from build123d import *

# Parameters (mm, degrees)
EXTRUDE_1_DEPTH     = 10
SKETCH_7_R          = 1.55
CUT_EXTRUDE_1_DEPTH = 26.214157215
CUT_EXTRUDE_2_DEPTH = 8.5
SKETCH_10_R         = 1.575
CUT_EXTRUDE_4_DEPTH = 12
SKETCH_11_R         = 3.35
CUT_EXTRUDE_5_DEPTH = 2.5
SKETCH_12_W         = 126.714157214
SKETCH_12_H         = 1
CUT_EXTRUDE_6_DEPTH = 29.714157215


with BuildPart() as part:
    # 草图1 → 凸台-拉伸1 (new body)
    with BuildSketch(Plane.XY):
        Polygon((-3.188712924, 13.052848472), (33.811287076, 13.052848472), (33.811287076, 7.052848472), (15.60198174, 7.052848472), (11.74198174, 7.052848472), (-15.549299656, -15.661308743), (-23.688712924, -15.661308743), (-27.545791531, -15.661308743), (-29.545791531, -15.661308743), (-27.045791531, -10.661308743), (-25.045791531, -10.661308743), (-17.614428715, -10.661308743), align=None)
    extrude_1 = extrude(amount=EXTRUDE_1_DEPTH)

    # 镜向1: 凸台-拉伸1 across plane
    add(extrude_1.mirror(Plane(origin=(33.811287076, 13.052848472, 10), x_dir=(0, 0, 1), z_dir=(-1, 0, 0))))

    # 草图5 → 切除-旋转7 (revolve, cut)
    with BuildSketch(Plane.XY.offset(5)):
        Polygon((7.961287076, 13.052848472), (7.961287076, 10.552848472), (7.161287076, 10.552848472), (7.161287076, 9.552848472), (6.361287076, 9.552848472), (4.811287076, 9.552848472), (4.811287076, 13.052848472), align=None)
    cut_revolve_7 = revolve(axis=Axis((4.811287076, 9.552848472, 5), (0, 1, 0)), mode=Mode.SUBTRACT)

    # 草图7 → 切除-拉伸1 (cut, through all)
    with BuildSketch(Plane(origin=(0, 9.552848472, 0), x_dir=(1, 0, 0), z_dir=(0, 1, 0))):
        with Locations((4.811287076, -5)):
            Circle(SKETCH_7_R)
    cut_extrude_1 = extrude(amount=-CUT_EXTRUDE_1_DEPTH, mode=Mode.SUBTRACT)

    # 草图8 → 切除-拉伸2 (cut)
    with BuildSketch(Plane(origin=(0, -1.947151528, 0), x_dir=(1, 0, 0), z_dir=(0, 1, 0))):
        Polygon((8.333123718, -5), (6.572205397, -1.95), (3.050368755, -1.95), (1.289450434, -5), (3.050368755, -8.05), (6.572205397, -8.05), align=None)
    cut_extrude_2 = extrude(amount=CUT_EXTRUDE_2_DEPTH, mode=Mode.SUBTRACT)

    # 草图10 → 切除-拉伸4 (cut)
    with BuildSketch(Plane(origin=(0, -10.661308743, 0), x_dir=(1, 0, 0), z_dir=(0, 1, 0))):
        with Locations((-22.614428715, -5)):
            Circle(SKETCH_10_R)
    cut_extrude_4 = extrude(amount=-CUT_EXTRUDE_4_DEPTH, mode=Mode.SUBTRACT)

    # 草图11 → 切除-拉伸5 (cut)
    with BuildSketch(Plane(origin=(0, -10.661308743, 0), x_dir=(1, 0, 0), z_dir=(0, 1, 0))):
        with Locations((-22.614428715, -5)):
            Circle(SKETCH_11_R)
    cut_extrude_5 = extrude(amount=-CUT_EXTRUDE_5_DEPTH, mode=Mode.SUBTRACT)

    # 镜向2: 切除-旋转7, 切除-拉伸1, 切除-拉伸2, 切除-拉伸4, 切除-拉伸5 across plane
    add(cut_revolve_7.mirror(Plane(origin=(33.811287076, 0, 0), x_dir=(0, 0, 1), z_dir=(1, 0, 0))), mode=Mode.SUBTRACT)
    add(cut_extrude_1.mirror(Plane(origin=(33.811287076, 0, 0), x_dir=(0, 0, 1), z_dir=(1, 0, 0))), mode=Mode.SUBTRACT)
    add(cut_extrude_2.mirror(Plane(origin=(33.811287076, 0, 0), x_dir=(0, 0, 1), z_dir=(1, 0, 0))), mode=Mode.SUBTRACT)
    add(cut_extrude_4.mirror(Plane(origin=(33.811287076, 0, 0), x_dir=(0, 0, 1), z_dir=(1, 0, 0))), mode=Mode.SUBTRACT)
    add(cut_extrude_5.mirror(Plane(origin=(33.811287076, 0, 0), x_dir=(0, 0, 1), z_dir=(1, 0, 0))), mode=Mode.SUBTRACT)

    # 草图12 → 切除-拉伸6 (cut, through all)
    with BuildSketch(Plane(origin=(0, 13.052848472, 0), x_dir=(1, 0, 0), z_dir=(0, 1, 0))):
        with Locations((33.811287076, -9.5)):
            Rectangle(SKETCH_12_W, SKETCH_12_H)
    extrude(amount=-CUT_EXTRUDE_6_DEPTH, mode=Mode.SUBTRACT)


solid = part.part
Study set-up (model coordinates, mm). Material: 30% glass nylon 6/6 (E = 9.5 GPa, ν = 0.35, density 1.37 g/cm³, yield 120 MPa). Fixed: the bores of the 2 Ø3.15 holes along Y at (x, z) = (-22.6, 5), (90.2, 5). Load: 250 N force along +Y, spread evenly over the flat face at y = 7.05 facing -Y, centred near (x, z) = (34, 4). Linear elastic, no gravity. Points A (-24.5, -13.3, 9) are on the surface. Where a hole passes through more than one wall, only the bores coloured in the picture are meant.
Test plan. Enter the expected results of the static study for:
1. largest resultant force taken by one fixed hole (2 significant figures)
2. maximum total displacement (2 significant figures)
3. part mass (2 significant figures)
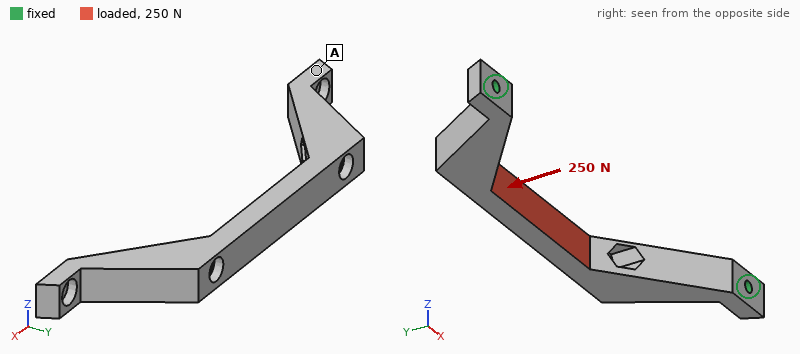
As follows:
230 N
0.17 mm
12 g
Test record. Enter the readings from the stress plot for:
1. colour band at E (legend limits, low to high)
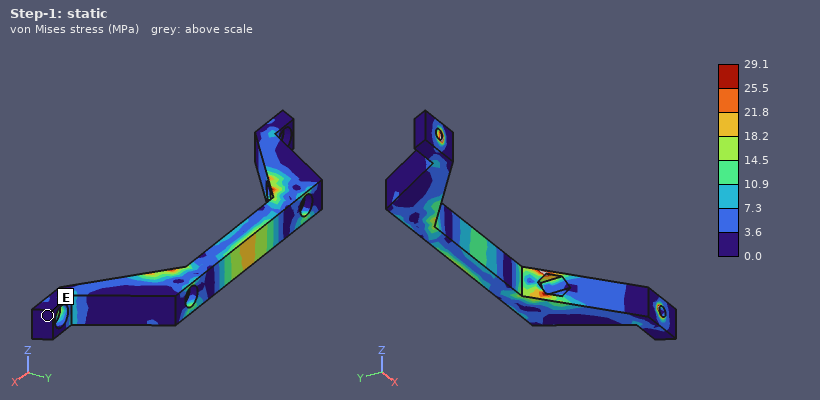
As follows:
0.0 to 3.6 MPa
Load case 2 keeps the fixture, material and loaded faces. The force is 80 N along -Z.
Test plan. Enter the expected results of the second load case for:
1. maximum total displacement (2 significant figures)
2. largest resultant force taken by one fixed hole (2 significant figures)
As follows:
0.54 mm
40 N
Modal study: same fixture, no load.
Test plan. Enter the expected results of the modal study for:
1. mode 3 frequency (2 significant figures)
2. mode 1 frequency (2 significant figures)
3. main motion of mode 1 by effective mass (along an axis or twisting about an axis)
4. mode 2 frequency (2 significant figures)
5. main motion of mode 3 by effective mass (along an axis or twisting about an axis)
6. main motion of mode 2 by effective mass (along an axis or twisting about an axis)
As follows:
2000 Hz
780 Hz
along Z
1800 Hz
twisting about Y
along X
